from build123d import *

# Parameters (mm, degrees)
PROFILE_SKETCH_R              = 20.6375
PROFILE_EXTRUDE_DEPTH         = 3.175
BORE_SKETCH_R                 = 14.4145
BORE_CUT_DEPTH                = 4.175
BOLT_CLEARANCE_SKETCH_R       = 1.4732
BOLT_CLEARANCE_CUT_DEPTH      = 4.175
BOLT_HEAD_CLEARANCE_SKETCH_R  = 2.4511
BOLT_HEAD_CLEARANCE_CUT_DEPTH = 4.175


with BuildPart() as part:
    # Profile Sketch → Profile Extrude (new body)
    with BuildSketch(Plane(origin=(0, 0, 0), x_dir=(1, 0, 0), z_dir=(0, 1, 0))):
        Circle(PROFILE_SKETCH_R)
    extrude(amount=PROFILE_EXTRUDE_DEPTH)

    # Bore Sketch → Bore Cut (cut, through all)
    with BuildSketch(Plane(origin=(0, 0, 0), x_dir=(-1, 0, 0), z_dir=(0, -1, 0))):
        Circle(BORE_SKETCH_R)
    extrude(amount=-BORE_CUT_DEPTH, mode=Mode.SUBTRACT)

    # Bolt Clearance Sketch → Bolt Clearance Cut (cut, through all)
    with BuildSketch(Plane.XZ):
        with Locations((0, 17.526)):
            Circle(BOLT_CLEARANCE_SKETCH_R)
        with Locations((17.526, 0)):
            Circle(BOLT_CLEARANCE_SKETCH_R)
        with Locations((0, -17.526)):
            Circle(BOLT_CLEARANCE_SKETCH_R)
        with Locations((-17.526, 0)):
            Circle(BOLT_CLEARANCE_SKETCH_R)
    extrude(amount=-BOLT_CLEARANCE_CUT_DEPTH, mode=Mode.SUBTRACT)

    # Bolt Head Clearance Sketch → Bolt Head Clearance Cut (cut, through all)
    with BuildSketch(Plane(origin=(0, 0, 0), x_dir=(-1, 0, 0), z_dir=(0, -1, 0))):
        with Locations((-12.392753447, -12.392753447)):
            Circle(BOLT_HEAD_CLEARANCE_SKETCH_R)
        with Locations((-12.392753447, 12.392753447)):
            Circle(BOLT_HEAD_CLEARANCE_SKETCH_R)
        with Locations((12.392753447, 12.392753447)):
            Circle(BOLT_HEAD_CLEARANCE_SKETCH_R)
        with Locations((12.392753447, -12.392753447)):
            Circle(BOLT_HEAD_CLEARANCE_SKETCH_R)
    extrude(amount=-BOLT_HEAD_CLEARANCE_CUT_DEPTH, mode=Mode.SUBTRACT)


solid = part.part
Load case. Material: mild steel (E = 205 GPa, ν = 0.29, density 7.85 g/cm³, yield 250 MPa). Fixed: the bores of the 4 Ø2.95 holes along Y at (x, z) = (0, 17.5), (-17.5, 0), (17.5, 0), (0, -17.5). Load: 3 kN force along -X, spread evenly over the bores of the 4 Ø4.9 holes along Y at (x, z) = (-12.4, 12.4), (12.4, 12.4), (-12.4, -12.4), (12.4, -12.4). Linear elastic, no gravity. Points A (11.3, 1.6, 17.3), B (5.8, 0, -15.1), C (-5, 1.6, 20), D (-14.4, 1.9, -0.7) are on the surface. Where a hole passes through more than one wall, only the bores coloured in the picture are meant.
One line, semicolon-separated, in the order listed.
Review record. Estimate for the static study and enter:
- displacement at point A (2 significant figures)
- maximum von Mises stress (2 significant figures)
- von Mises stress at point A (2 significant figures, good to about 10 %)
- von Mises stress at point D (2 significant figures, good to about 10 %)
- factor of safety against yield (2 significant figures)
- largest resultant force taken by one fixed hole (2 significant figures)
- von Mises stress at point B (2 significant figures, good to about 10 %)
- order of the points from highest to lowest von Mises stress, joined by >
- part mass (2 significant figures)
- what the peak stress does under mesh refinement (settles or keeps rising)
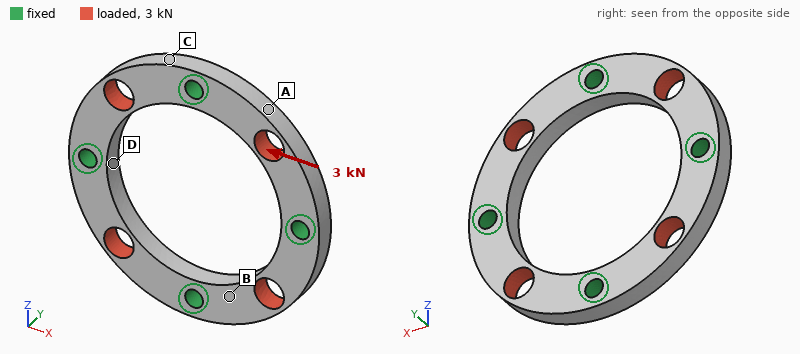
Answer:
2.0 µm; 200 MPa; 55 MPa; 84 MPa; 1.2; 1.1 kN; 33 MPa; D > A > B > C; 15 g; settles
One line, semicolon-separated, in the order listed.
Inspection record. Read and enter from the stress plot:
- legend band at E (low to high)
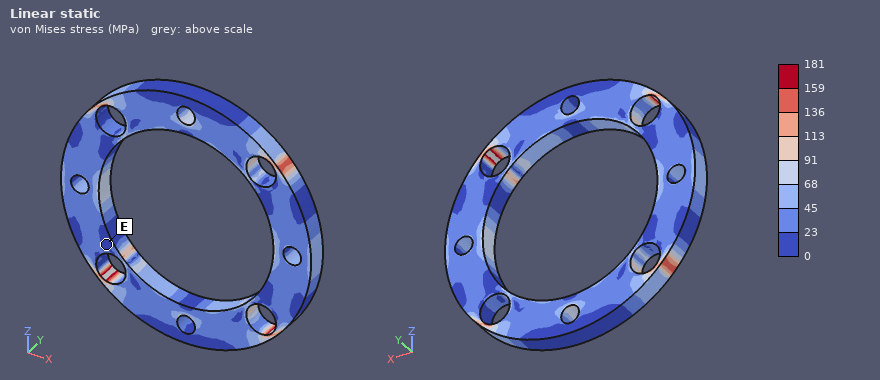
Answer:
0 to 23 MPa
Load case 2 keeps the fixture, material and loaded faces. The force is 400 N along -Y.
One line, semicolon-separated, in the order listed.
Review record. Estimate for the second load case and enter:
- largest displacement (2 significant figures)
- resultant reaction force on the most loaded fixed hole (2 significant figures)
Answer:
6.0 µm; 100 N
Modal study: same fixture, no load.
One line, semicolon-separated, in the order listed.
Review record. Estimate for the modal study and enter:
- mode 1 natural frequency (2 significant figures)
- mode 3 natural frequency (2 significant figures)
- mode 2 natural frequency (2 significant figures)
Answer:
22 kHz; 22 kHz; 22 kHz
